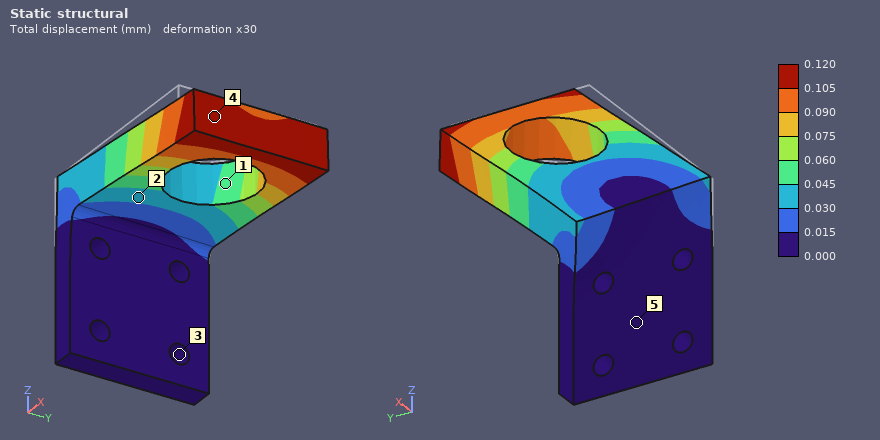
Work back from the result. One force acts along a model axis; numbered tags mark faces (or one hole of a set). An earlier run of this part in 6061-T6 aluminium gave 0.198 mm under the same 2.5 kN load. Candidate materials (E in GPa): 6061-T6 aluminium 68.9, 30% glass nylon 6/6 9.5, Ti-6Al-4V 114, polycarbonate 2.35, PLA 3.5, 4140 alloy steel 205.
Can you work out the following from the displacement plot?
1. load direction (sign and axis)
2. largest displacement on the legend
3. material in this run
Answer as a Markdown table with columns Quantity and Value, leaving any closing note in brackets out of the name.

| Quantity | Value |
|---|---|
| load direction | +Y |
| largest displacement on the legend | 0.120 mm |
| material in this run | Ti-6Al-4V |
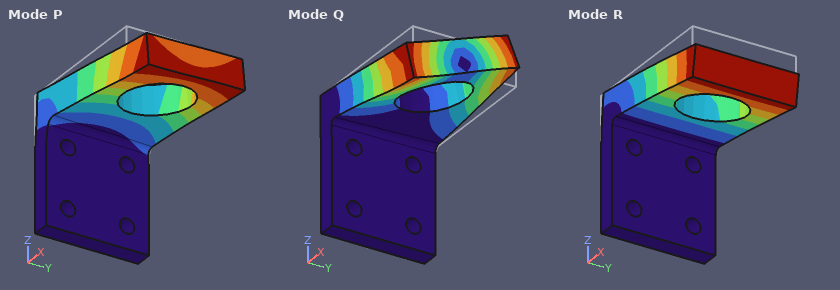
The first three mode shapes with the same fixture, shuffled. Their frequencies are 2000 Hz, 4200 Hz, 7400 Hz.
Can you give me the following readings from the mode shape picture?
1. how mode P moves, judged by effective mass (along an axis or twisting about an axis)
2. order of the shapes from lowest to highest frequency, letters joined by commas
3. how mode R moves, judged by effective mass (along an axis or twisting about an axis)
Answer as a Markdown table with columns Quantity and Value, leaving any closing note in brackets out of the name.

| Quantity | Value |
|---|---|
| how mode P moves, judged by effective mass | along Y |
| order of the shapes from lowest to highest frequency, letters joined by commas | R, P, Q |
| how mode R moves, judged by effective mass | along Z |
